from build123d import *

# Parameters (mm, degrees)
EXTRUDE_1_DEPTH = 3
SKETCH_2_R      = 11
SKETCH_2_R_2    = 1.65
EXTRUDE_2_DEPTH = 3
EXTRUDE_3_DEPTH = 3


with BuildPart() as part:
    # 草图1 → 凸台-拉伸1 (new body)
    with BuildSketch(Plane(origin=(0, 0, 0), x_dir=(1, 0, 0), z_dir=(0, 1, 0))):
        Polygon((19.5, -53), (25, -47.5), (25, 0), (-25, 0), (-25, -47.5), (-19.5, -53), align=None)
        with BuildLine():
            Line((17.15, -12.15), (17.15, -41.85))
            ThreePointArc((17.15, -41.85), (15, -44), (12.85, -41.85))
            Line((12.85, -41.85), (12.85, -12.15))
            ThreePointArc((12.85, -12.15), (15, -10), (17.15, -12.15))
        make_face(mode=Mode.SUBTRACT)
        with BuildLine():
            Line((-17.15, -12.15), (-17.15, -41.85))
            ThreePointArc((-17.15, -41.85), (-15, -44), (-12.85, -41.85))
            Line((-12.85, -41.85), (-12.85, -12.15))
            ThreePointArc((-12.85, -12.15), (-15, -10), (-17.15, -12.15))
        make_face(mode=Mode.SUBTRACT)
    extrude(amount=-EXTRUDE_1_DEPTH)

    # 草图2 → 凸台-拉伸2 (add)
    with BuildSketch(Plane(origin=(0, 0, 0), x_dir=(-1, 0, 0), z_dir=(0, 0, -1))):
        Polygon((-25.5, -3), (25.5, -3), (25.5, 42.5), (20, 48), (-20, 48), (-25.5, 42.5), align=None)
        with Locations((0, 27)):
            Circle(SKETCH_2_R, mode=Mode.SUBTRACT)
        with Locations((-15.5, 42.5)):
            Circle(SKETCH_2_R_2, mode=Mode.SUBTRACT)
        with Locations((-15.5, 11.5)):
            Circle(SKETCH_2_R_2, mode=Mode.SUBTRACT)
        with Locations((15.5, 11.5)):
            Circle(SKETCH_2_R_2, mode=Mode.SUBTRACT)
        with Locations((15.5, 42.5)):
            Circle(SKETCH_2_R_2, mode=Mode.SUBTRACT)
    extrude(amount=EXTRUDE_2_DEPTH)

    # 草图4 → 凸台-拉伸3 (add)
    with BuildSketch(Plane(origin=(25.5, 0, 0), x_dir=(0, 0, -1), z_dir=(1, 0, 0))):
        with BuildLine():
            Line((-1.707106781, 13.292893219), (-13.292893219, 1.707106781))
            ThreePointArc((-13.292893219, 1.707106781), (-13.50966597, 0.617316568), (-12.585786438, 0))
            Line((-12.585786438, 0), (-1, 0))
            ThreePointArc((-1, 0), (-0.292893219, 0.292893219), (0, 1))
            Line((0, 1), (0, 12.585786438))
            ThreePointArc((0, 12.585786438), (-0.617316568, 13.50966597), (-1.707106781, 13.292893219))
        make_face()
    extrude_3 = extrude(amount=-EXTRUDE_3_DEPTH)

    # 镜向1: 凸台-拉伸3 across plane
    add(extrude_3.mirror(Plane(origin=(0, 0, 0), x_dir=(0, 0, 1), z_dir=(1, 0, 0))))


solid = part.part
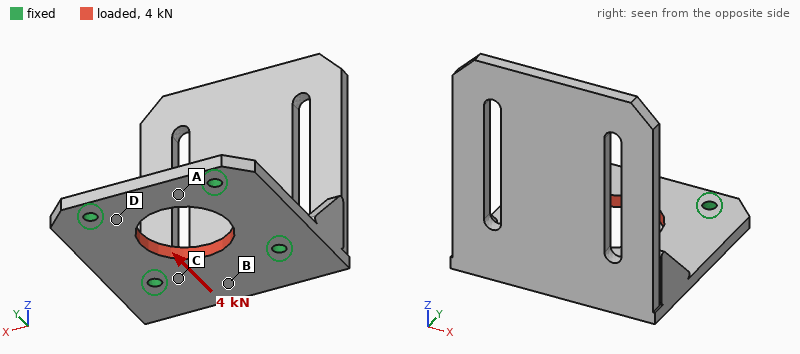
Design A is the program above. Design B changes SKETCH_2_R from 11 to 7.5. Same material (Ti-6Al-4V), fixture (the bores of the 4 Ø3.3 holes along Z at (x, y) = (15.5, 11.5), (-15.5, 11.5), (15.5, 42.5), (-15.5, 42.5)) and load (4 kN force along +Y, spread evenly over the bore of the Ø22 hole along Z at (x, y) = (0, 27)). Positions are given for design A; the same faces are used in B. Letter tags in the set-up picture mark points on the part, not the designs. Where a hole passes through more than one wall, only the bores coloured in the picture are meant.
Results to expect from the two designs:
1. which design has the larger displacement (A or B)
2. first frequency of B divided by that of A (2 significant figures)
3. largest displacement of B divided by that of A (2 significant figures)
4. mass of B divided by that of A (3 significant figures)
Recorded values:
A
1.0
0.91
1.04
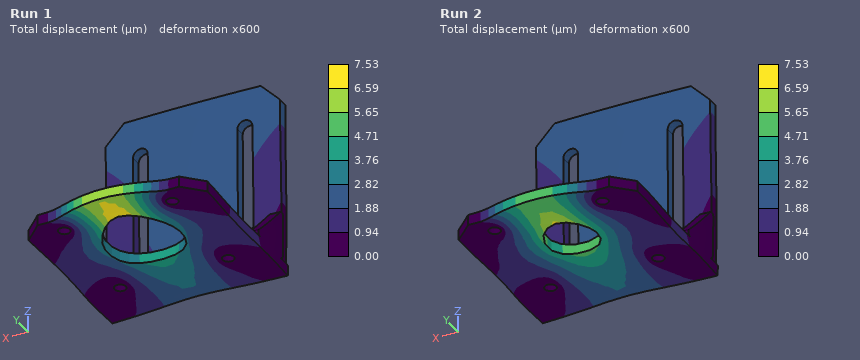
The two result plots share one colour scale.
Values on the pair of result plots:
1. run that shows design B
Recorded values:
Run 2
